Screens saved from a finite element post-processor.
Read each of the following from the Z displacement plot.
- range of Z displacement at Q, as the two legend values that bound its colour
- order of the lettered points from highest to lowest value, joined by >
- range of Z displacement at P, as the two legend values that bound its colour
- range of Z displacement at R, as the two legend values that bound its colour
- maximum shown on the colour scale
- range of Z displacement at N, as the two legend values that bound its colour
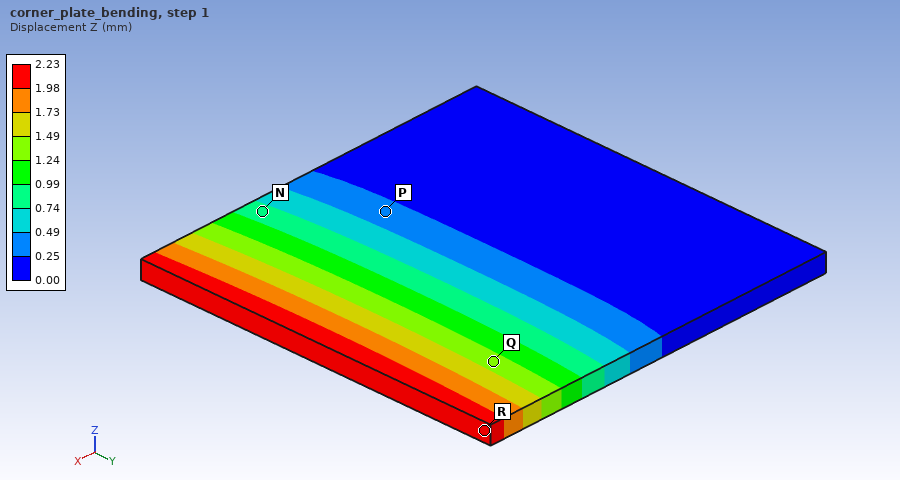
1.24 to 1.49 mm
R > Q > N > P
0.25 to 0.49 mm
1.98 to 2.23 mm
2.23 mm
0.74 to 0.99 mm
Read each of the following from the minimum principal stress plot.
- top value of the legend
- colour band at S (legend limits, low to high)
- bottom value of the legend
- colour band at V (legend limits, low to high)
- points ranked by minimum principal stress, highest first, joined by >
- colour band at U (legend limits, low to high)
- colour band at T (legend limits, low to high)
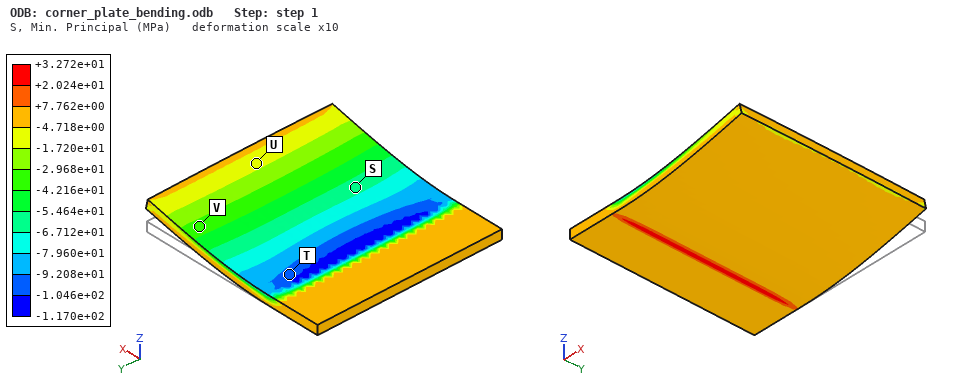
+3.272e+01 MPa
-6.712e+01 to -5.464e+01 MPa
-1.170e+02 MPa
-4.216e+01 to -2.968e+01 MPa
U > V > S > T
-1.720e+01 to -4.718e+00 MPa
-1.046e+02 to -9.208e+01 MPa
